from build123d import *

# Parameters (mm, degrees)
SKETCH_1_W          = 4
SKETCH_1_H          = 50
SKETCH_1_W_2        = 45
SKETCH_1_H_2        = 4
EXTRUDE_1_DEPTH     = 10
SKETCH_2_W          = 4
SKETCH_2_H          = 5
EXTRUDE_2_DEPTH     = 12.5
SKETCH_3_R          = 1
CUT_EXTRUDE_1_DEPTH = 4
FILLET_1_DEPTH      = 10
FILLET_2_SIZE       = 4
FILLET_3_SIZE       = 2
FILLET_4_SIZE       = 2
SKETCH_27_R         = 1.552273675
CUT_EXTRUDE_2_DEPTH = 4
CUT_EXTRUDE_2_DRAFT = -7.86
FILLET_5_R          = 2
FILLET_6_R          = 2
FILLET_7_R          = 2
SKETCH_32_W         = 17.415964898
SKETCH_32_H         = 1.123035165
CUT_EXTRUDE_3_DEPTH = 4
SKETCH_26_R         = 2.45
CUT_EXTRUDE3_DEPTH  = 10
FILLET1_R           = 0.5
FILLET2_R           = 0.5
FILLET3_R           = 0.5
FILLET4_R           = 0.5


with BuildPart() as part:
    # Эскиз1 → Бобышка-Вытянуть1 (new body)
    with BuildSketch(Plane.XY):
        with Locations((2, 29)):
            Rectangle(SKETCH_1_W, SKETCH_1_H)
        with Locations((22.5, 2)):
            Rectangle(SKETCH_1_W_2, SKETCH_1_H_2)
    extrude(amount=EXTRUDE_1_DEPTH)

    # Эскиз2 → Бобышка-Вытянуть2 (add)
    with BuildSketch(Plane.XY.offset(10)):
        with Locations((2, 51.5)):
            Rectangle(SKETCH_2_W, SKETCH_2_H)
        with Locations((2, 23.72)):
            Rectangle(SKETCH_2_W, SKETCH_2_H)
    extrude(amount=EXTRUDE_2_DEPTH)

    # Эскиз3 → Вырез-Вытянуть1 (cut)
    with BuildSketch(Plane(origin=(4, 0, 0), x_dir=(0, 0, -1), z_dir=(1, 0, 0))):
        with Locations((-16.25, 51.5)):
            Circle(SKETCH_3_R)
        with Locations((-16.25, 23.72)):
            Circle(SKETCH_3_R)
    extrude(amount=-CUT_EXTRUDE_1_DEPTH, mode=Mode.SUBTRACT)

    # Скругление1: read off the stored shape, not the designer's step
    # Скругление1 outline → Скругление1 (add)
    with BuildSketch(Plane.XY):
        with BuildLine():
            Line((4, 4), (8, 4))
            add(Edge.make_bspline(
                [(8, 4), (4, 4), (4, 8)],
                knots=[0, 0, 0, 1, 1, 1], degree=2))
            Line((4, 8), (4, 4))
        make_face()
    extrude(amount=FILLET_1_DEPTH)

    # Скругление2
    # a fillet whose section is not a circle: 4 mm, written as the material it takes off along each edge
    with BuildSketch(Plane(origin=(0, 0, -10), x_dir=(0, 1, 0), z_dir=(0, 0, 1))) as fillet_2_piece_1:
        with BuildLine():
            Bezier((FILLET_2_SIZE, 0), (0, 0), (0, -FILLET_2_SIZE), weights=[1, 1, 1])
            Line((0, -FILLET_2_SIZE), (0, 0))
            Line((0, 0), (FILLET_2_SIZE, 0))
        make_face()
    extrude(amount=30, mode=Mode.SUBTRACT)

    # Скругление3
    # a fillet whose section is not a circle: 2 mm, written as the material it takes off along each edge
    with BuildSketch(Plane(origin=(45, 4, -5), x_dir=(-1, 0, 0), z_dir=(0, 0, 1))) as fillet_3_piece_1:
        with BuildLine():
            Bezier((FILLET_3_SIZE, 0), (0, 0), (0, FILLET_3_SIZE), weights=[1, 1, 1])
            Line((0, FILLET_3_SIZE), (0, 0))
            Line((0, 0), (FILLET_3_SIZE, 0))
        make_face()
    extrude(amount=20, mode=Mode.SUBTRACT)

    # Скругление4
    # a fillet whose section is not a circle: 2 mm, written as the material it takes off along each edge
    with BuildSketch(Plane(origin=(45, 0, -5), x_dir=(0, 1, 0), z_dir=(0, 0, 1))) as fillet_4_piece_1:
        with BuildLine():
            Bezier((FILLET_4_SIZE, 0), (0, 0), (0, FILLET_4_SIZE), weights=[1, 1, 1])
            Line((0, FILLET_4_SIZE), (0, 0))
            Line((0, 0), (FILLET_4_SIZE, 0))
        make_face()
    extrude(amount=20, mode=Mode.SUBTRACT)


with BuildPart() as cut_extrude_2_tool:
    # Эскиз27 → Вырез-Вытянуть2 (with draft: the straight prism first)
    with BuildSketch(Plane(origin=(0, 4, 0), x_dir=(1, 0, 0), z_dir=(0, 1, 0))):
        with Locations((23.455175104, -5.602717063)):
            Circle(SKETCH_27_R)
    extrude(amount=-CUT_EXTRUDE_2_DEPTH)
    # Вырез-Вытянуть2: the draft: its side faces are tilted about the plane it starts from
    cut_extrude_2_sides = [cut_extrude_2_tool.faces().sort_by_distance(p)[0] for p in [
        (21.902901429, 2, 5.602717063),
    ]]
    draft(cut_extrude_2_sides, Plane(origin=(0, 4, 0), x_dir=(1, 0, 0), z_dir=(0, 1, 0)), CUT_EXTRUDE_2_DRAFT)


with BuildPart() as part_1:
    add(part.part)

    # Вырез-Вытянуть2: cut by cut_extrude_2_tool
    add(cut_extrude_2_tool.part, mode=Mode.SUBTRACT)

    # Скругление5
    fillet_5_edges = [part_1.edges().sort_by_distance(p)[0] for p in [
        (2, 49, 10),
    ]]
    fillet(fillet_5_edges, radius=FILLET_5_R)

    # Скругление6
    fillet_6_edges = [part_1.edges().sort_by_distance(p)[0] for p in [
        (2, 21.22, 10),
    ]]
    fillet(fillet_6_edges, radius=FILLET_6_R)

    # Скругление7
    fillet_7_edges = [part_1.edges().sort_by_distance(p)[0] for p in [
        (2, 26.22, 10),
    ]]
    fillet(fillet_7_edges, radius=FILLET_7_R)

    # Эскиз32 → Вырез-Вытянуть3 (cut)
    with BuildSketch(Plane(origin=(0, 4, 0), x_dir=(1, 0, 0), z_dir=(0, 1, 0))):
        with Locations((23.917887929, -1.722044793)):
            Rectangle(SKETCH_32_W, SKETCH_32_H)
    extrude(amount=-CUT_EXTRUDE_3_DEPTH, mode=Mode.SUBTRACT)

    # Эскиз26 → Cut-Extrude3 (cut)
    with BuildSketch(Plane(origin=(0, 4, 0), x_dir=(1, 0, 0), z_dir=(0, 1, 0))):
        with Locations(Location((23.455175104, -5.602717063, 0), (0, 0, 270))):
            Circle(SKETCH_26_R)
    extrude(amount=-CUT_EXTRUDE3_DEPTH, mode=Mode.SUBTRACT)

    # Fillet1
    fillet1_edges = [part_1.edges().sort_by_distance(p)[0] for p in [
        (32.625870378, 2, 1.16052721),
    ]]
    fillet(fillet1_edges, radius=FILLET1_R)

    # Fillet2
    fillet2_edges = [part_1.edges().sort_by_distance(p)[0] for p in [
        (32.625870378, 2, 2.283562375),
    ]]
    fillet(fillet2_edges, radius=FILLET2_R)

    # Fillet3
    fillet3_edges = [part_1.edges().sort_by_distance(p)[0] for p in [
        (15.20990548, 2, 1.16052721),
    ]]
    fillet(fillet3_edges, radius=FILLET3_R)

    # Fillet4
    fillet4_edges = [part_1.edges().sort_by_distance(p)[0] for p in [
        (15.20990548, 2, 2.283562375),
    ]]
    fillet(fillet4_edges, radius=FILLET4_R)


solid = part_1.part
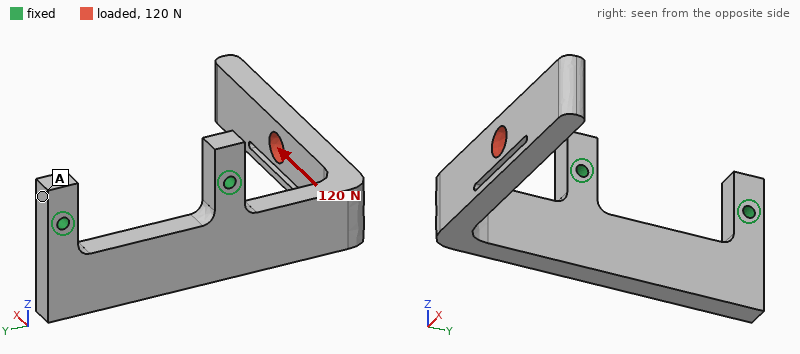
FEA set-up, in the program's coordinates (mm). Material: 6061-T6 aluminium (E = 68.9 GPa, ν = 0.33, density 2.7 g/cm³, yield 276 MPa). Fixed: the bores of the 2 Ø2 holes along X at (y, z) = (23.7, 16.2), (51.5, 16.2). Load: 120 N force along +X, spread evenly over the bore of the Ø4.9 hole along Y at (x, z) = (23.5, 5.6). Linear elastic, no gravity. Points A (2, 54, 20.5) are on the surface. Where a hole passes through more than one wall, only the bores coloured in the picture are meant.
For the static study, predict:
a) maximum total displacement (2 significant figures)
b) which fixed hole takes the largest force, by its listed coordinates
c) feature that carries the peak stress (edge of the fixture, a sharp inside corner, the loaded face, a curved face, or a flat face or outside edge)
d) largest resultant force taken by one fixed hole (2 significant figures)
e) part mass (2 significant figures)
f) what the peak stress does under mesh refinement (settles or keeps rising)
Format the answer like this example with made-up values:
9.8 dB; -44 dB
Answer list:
0.59 mm; (23.7, 16.2); edge of the fixture; 180 N; 11 g; keeps rising
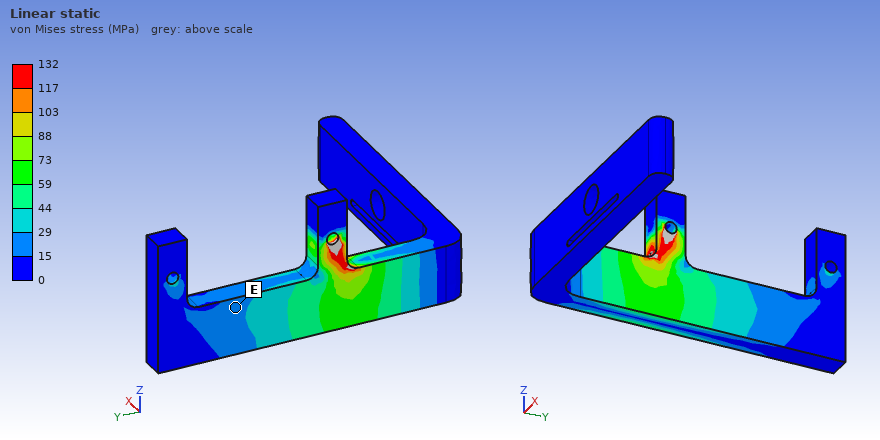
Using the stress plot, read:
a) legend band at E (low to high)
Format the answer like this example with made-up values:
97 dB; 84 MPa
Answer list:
15 to 29 MPa
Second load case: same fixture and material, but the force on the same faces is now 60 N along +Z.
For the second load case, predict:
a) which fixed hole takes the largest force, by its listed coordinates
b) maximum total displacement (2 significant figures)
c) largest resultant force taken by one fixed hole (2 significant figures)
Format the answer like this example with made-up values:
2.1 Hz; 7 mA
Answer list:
(23.7, 16.2); 0.45 mm; 110 N
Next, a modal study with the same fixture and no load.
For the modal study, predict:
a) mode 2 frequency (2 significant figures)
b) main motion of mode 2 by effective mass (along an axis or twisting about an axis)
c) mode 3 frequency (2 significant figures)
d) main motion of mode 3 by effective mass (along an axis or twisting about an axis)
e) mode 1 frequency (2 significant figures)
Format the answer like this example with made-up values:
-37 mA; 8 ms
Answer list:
1100 Hz; along Z; 2700 Hz; along X; 900 Hz
